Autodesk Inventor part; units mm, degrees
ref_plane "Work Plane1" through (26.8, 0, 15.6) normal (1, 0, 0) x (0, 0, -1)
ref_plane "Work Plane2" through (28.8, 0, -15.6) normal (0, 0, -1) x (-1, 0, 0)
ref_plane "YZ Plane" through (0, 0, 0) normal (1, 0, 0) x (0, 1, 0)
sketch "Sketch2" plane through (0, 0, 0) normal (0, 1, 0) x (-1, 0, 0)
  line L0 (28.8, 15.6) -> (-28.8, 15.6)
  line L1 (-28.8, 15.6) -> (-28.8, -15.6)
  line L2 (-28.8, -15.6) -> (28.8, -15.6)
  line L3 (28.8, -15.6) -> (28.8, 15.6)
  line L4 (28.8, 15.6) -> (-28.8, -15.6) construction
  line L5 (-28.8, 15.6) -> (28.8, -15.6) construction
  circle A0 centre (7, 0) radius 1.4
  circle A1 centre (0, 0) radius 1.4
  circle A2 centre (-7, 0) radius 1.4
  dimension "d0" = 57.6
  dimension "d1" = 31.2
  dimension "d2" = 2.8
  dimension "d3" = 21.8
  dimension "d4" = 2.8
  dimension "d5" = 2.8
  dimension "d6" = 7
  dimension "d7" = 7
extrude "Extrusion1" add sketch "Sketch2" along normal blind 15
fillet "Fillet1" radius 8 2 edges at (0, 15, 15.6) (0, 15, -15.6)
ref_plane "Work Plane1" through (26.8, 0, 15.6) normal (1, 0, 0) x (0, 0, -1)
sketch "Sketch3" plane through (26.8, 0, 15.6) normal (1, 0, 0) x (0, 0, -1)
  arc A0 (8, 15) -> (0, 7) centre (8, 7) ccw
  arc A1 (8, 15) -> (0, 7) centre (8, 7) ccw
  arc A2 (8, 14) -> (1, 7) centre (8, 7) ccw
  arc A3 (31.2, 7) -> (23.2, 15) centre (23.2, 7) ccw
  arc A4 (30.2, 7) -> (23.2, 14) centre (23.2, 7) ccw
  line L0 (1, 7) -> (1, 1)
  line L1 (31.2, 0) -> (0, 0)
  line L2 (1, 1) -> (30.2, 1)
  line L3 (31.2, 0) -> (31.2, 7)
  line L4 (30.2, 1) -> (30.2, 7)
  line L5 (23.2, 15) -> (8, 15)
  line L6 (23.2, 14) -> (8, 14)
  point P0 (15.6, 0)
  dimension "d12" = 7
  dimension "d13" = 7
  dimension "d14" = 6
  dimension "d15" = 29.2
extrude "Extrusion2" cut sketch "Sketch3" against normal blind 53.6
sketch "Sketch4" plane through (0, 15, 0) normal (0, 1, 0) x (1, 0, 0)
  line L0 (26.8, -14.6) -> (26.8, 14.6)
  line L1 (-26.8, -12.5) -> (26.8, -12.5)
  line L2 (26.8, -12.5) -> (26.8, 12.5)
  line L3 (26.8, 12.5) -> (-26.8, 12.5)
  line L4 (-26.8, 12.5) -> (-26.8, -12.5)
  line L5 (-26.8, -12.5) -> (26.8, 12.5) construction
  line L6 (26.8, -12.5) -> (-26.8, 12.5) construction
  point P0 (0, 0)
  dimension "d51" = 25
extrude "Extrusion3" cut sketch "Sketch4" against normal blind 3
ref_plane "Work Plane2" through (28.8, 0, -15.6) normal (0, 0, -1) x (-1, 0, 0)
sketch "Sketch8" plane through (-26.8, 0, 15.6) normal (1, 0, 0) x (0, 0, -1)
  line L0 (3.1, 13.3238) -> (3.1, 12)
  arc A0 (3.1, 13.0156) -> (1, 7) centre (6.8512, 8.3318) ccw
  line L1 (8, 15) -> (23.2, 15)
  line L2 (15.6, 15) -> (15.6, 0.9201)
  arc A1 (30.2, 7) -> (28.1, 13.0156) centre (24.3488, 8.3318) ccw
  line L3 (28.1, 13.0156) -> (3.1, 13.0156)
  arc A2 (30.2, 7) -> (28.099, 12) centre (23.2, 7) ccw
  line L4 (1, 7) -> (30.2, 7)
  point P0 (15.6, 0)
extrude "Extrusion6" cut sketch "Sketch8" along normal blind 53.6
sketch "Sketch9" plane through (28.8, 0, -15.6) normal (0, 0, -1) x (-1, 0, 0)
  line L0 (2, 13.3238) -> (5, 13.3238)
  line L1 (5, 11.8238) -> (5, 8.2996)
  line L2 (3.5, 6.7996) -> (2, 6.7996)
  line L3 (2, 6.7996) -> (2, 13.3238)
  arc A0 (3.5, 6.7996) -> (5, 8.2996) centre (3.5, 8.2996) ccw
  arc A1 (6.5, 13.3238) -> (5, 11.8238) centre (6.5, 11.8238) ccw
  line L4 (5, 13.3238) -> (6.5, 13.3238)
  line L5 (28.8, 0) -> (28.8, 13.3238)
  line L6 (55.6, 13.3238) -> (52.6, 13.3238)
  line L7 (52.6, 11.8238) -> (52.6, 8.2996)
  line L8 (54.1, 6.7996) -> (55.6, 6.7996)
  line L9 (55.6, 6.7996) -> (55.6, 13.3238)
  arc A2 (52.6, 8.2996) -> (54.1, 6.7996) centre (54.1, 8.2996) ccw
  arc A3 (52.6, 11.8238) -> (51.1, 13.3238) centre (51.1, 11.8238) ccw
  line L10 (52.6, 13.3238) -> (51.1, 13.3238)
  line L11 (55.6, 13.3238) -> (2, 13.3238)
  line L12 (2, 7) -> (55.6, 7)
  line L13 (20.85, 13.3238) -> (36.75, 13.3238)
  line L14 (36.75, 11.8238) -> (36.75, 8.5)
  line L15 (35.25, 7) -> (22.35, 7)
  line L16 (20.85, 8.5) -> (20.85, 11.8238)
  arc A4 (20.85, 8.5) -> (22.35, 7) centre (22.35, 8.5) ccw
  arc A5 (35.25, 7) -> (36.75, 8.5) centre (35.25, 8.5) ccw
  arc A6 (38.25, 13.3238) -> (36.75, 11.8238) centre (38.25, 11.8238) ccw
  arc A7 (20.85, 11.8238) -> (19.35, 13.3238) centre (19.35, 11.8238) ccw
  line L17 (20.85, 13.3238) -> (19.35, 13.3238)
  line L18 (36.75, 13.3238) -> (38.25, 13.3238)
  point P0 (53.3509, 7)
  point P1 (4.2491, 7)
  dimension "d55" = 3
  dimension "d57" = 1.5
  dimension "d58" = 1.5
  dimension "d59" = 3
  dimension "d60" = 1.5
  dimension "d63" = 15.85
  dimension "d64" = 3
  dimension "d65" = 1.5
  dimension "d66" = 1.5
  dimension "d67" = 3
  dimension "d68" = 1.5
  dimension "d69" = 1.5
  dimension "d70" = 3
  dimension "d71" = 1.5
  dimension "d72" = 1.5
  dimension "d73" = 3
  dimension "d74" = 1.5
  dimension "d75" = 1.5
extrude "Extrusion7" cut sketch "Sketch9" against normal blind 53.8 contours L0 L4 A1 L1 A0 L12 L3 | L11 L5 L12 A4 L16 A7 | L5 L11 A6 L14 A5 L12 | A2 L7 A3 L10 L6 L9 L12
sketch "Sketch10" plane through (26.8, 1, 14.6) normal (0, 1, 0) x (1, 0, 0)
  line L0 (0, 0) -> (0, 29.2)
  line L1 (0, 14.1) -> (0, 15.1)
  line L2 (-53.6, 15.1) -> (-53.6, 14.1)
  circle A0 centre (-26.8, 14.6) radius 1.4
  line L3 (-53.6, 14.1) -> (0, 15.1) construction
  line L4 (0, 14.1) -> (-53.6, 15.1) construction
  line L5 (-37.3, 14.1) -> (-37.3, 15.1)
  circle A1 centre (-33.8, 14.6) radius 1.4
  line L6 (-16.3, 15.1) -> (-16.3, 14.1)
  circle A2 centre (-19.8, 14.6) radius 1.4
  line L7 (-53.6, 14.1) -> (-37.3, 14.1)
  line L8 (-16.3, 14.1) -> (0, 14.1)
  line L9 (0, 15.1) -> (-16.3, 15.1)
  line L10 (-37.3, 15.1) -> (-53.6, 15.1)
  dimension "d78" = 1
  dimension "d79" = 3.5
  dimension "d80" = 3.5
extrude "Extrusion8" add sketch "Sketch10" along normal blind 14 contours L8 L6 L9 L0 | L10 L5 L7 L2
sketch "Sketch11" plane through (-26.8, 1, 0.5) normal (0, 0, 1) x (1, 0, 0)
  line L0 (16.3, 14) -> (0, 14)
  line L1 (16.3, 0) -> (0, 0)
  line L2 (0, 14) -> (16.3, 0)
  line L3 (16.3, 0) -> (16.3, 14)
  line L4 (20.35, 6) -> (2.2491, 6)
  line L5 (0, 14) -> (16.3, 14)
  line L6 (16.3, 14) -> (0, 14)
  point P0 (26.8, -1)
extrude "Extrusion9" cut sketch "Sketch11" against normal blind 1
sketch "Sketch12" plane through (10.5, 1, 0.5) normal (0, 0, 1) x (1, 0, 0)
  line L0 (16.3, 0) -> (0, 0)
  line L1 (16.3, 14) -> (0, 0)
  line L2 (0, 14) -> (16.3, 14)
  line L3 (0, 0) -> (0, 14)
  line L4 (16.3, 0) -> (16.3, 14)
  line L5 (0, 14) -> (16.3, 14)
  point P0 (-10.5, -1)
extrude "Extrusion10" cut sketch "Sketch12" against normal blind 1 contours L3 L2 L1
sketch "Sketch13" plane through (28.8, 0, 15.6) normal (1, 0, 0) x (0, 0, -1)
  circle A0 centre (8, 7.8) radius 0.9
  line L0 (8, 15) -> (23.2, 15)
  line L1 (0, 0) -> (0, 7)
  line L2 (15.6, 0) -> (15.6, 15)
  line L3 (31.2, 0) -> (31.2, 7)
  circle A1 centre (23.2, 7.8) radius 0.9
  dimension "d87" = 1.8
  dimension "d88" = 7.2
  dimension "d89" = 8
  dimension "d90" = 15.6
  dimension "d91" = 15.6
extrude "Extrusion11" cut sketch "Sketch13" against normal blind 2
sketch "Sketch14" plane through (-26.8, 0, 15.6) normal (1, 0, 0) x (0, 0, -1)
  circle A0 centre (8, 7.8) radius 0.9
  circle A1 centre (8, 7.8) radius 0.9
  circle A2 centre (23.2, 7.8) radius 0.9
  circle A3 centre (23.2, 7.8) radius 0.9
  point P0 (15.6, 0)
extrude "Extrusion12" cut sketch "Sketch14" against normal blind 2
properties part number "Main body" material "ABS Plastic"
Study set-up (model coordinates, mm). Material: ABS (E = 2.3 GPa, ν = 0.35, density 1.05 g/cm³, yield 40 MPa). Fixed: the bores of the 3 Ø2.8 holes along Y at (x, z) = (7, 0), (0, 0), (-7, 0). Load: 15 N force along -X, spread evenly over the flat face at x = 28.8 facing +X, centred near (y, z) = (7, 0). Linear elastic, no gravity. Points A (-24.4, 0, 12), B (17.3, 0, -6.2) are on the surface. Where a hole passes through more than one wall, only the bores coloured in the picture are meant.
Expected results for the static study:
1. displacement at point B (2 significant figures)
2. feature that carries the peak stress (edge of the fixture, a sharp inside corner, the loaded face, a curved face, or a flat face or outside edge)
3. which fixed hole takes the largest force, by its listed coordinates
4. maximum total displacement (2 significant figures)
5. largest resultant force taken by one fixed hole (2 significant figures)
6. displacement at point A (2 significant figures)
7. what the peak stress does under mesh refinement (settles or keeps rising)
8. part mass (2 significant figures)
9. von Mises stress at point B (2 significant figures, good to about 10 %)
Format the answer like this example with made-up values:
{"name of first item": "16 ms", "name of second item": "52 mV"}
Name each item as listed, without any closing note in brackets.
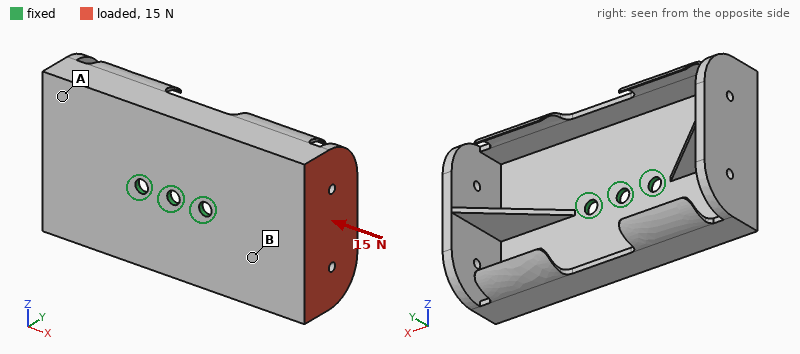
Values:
{"displacement at point B": "0.26 mm", "feature that carries the peak stress": "edge of the fixture", "which fixed hole takes the largest force, by its listed coordinates": "(7, 0)", "maximum total displacement": "0.74 mm", "largest resultant force taken by one fixed hole": "8.3 N", "displacement at point A": "0.32 mm", "what the peak stress does under mesh refinement": "keeps rising", "part mass": "4.7 g", "von Mises stress at point B": "2.1 MPa"}
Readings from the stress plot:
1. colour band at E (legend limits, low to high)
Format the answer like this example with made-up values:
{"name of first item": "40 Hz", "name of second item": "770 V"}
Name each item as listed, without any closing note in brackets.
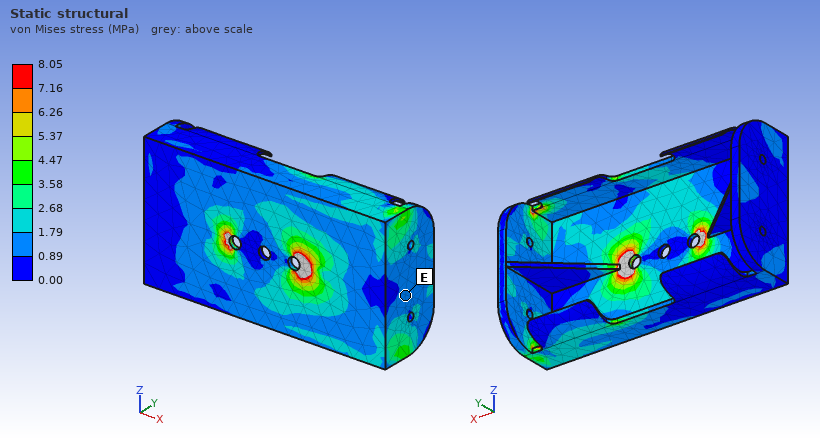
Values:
{"colour band at E": "0.89 to 1.79 MPa"}
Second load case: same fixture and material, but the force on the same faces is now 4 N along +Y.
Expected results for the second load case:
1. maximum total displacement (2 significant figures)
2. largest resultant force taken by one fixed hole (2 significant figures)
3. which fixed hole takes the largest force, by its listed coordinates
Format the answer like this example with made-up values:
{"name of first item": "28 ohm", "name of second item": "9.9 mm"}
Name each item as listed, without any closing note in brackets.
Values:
{"maximum total displacement": "0.65 mm", "largest resultant force taken by one fixed hole": "7.9 N", "which fixed hole takes the largest force, by its listed coordinates": "(7, 0)"}
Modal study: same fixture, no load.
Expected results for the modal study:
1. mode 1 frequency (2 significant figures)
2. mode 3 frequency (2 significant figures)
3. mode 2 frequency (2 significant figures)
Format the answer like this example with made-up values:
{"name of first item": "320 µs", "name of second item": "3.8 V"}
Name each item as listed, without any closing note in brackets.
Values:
{"mode 1 frequency": "300 Hz", "mode 3 frequency": "460 Hz", "mode 2 frequency": "350 Hz"}
